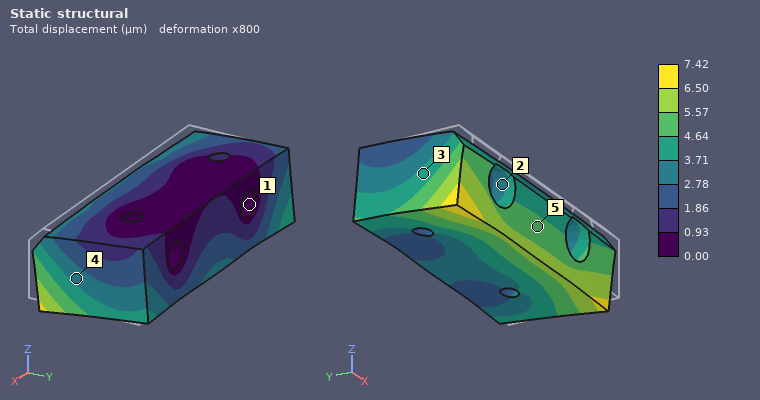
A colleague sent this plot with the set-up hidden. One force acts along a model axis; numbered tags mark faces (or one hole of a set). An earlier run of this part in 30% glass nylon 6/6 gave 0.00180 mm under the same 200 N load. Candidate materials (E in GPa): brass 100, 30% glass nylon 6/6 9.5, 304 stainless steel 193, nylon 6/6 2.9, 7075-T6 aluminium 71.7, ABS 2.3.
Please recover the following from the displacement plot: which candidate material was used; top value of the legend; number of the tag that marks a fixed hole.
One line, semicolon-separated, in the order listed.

ABS; 7.42 µm; 1
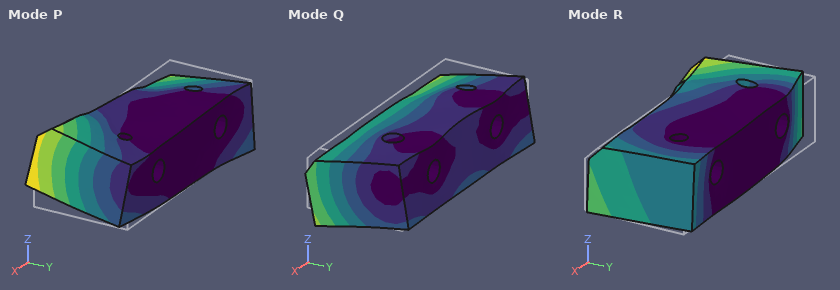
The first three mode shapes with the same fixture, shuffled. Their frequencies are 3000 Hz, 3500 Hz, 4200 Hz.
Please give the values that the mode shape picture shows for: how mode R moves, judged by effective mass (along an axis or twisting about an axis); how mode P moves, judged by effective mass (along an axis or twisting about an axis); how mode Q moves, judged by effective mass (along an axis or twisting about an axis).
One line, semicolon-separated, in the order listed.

along X; twisting about Y; along Z
